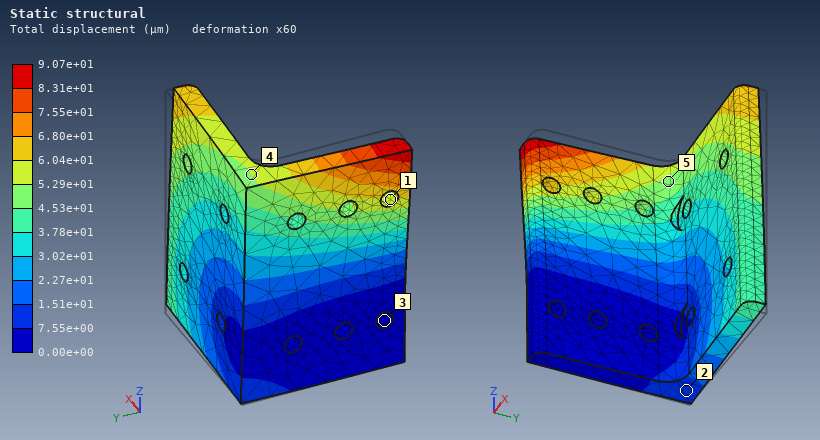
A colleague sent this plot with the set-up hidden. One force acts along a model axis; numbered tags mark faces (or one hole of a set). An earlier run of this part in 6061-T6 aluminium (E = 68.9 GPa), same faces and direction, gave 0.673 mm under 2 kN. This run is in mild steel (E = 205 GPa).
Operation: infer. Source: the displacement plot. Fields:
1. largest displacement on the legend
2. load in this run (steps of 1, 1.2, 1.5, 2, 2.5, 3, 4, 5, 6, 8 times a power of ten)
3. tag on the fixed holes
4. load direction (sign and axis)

9.07e+01 µm
800 N
3
-X
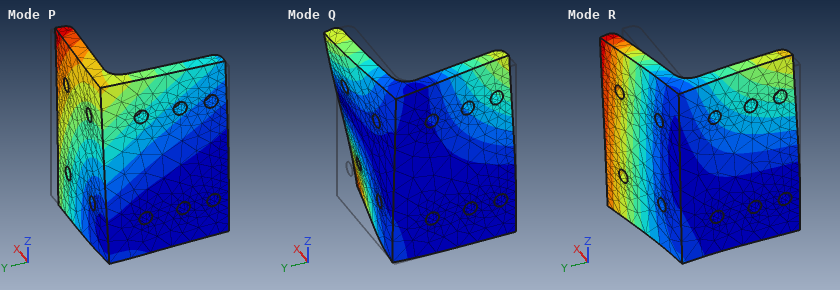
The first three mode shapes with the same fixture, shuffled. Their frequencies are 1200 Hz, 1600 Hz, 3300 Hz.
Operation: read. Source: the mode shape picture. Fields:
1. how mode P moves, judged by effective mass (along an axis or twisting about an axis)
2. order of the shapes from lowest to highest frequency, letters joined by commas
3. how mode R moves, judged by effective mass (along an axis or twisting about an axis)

along X
P, R, Q
along Y
